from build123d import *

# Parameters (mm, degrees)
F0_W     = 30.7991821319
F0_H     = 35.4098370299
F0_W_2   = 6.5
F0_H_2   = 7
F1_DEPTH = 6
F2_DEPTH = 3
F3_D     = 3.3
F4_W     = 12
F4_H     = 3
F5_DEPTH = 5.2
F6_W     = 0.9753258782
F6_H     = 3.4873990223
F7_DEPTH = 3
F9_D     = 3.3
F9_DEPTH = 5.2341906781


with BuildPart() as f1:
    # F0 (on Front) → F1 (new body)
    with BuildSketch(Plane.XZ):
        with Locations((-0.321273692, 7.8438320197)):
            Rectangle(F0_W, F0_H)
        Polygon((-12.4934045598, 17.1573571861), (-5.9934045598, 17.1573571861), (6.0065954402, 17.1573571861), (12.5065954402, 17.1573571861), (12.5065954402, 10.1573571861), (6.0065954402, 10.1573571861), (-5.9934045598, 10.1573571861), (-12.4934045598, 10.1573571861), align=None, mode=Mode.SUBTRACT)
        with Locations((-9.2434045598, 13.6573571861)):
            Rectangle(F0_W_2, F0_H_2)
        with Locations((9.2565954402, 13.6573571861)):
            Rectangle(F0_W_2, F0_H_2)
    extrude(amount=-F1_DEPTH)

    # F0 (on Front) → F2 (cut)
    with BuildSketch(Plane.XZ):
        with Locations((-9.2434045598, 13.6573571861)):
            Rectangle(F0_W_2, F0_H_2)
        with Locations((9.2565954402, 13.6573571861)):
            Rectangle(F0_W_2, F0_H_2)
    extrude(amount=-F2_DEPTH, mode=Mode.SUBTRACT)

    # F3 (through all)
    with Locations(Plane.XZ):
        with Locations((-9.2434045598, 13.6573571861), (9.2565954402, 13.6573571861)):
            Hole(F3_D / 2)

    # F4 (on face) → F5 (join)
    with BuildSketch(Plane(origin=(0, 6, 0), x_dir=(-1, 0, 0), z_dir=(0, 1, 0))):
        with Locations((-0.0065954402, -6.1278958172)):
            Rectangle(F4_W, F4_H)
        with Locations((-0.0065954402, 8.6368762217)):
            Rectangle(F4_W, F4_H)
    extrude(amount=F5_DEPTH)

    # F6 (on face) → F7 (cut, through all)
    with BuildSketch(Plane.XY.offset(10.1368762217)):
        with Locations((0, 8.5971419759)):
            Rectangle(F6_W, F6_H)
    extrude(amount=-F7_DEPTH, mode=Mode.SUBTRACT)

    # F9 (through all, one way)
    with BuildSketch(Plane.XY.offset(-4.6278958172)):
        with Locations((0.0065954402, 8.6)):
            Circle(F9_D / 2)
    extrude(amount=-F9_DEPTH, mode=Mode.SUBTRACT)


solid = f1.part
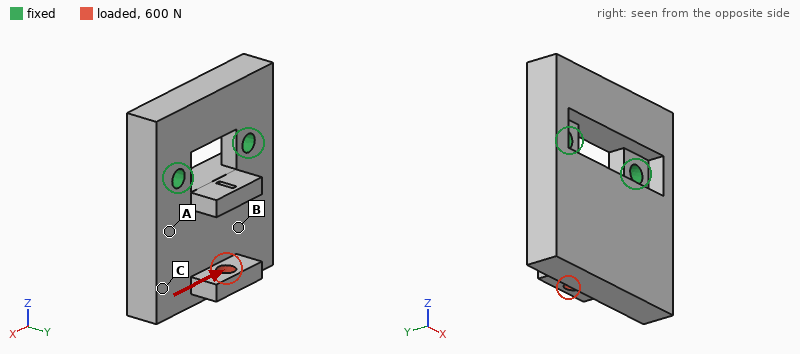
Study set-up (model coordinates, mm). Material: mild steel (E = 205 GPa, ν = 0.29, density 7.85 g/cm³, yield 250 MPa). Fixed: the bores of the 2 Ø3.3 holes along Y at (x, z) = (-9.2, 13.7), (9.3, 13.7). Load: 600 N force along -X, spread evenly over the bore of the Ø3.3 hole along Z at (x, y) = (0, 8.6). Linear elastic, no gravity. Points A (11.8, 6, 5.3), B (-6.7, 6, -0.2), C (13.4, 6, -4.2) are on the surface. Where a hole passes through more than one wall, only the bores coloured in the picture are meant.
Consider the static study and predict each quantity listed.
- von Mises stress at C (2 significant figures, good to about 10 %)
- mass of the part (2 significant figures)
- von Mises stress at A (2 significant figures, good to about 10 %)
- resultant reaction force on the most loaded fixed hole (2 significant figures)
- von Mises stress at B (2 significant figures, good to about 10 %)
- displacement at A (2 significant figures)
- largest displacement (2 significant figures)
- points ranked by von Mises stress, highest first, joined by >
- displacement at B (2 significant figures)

7.4 MPa
48 g
16 MPa
620 N
24 MPa
2.8 µm
9.1 µm
B > A > C
3.5 µm
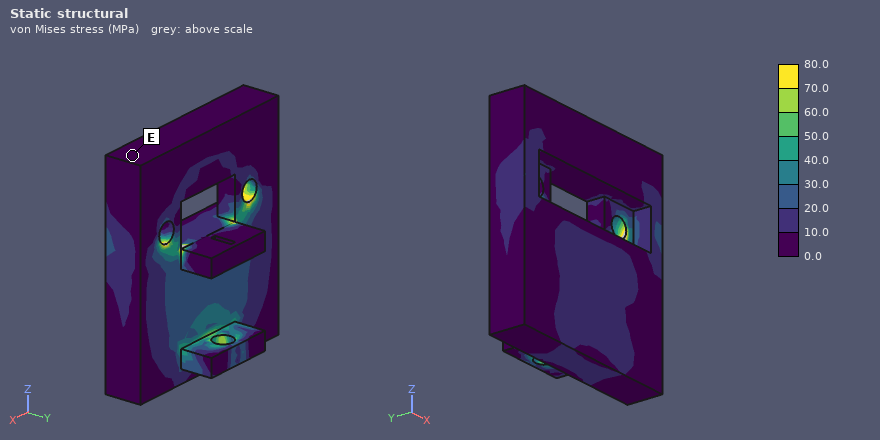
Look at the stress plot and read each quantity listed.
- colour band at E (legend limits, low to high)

0.0 to 10.0 MPa
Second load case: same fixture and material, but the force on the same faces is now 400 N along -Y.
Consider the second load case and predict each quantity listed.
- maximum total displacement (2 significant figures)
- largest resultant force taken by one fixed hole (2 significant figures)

47 µm
210 N
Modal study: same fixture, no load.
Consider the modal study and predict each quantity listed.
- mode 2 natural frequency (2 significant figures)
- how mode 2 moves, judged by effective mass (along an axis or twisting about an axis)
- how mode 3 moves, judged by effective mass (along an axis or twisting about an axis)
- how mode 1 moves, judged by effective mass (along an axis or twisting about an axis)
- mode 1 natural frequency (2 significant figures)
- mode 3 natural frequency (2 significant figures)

12 kHz
twisting about Z
along Y
along Y
4000 Hz
14 kHz
